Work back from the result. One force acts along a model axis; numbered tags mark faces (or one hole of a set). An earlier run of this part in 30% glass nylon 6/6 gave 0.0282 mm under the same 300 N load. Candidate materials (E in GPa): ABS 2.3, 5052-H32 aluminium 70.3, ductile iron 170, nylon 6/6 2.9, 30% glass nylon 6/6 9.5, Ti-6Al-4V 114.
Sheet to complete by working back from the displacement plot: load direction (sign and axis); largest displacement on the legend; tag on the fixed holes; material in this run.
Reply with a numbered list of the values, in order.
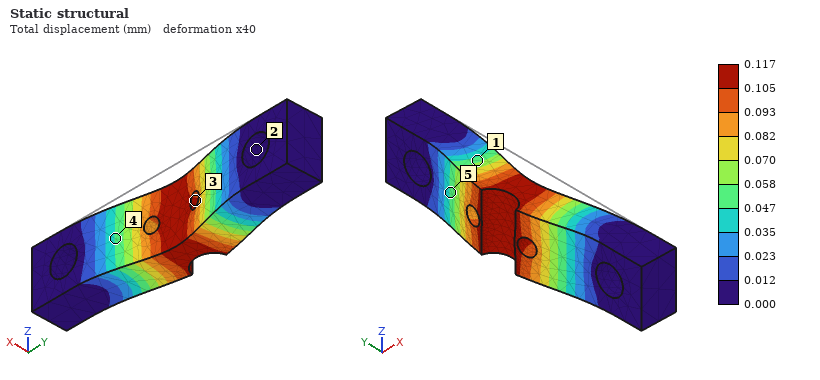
1. -X
2. 0.117 mm
3. 2
4. ABS
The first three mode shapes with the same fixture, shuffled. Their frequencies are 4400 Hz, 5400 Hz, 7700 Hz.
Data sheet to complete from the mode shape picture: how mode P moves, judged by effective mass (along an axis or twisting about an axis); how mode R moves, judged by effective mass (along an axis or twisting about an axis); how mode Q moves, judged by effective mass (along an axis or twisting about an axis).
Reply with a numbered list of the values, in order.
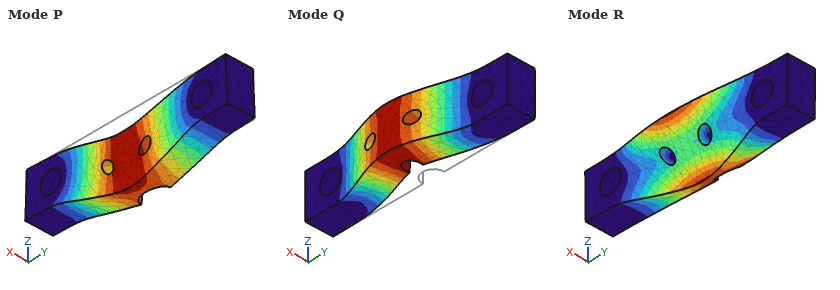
1. along Z
2. twisting about Y
3. along X
